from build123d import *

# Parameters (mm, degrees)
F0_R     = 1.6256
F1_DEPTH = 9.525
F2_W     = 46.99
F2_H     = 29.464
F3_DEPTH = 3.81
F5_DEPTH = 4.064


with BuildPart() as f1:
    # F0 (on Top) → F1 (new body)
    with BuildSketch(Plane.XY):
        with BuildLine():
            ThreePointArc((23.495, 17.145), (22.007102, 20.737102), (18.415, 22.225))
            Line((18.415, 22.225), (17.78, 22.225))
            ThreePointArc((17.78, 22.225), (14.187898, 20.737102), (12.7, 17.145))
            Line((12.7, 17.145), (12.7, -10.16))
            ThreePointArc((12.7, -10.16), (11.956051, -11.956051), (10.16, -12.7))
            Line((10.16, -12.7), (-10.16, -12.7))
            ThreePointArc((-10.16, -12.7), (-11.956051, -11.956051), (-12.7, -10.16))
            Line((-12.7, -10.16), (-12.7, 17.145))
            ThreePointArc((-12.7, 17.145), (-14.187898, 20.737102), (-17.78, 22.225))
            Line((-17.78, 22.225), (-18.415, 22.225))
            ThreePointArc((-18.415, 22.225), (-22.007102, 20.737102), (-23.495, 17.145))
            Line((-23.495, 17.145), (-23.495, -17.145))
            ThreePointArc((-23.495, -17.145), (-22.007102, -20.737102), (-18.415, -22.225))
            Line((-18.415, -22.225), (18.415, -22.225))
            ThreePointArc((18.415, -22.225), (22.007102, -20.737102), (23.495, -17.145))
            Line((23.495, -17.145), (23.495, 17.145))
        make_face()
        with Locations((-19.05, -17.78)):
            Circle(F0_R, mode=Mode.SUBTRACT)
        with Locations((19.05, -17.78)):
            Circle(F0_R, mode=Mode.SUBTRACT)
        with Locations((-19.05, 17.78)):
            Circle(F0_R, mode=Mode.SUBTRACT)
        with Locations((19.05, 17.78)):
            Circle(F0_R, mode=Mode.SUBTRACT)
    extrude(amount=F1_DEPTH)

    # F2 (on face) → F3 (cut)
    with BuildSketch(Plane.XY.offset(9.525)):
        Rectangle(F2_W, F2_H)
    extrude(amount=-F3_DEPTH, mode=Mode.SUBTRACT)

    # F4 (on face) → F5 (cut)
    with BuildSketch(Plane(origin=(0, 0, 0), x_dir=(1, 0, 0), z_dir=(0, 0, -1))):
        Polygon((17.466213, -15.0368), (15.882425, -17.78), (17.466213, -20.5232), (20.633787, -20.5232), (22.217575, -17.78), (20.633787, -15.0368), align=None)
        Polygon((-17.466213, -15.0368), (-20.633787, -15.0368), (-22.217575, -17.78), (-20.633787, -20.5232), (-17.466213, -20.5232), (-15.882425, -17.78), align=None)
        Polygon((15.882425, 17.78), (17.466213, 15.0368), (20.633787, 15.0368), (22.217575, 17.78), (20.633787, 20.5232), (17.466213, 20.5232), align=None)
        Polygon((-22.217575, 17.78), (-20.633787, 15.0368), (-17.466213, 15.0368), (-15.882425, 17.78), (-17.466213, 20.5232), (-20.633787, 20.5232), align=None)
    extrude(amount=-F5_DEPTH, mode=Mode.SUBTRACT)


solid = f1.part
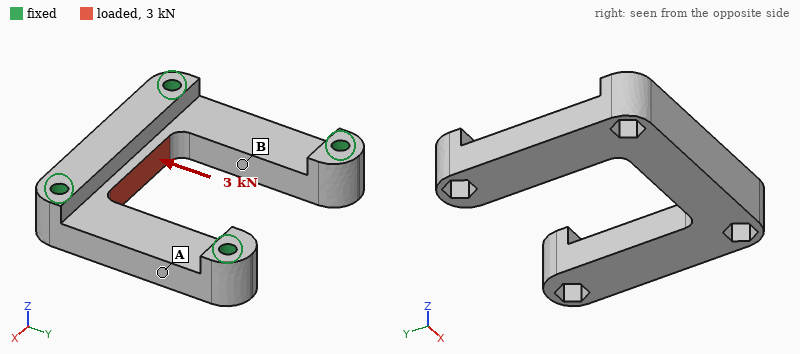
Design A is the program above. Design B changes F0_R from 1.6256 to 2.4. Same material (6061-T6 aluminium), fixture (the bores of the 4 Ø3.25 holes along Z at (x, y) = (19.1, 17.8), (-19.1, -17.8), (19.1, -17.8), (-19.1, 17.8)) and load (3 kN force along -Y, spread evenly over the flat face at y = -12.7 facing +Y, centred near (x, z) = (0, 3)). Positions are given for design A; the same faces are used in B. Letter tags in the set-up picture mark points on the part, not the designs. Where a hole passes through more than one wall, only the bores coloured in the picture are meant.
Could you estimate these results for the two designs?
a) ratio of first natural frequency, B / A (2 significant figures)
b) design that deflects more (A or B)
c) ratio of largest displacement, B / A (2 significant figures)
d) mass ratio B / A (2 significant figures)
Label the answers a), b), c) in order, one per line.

a) 1.1
b) A
c) 0.88
d) 0.97
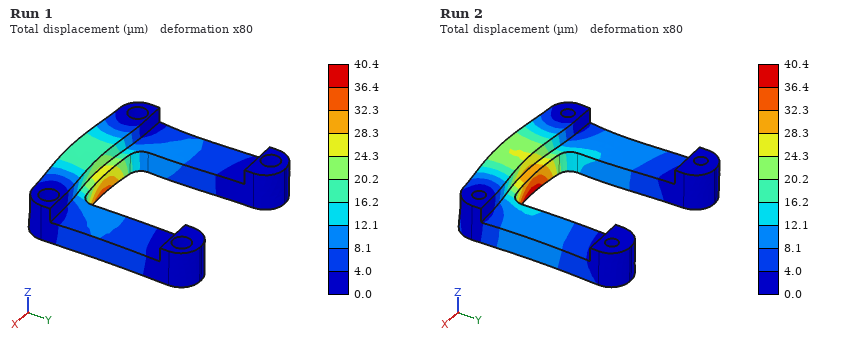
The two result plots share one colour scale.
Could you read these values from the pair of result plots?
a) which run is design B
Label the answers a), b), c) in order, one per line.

a) Run 1
